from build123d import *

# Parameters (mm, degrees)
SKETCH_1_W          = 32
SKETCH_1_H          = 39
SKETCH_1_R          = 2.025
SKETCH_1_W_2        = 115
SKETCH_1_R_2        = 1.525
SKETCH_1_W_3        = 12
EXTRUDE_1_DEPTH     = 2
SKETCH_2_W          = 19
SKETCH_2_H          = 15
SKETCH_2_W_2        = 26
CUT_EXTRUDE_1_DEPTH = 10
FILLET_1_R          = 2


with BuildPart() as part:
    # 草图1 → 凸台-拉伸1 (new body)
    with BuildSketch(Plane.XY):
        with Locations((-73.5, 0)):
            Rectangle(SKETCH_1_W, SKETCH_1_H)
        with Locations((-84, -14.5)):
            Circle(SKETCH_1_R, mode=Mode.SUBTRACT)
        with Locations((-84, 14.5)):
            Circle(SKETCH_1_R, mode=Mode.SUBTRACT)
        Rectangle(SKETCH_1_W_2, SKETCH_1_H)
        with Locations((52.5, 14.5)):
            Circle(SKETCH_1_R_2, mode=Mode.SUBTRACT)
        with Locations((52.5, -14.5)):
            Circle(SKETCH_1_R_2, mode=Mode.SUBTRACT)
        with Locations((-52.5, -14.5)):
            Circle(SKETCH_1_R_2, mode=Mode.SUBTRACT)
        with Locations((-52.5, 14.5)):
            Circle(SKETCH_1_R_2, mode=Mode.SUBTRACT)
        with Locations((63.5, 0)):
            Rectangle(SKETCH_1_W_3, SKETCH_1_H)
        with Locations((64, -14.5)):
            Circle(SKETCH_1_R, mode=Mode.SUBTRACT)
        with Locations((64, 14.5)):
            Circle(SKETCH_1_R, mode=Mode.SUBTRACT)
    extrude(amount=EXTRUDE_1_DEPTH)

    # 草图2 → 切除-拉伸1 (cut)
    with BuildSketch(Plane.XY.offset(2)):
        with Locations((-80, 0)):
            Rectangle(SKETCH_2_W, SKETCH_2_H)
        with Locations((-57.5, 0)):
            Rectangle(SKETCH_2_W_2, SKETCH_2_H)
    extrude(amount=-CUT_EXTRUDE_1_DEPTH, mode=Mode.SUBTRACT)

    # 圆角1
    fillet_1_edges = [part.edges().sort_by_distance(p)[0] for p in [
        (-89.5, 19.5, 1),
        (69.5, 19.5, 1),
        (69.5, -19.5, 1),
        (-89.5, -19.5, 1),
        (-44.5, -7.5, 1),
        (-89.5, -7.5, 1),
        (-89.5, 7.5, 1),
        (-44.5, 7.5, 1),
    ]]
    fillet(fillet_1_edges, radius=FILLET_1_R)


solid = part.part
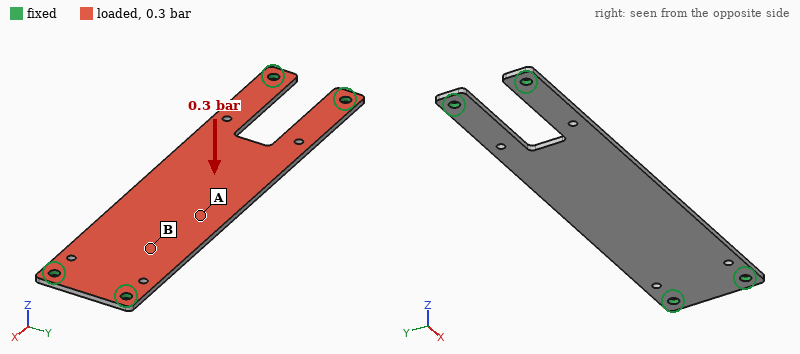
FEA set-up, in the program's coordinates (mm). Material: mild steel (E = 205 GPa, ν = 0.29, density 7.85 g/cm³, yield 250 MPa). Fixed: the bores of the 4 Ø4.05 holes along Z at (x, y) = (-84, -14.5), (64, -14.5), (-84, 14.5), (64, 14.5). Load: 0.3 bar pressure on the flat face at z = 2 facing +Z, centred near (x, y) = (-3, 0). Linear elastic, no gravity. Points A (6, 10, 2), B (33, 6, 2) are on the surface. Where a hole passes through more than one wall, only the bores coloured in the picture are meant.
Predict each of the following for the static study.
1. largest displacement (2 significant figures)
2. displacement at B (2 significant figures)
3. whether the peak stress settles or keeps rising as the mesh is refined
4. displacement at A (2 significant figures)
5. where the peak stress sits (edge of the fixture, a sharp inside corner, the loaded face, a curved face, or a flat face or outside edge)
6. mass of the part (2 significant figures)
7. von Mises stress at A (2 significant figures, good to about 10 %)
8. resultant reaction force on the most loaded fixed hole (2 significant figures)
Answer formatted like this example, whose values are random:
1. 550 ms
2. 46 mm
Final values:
1. 0.30 mm
2. 0.13 mm
3. keeps rising
4. 0.26 mm
5. edge of the fixture
6. 85 g
7. 35 MPa
8. 46 N
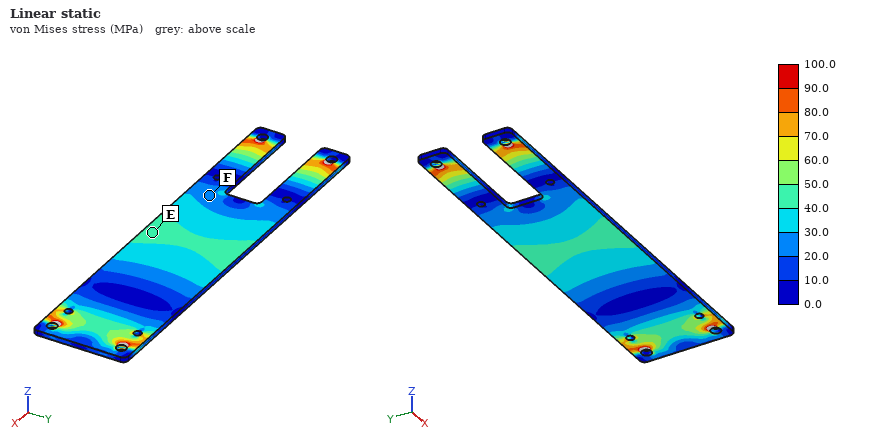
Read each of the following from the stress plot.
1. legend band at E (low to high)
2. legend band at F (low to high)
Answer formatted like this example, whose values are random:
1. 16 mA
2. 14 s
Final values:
1. 40.0 to 50.0 MPa
2. 20.0 to 30.0 MPa
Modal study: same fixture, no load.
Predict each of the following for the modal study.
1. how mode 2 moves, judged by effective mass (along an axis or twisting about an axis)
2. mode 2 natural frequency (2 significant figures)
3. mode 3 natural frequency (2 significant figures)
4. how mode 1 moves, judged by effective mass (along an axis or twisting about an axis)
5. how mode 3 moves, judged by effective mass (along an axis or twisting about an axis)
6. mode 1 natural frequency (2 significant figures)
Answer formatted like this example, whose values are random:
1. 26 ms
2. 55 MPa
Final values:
1. twisting about X
2. 1200 Hz
3. 1300 Hz
4. along Z
5. twisting about Y
6. 460 Hz
